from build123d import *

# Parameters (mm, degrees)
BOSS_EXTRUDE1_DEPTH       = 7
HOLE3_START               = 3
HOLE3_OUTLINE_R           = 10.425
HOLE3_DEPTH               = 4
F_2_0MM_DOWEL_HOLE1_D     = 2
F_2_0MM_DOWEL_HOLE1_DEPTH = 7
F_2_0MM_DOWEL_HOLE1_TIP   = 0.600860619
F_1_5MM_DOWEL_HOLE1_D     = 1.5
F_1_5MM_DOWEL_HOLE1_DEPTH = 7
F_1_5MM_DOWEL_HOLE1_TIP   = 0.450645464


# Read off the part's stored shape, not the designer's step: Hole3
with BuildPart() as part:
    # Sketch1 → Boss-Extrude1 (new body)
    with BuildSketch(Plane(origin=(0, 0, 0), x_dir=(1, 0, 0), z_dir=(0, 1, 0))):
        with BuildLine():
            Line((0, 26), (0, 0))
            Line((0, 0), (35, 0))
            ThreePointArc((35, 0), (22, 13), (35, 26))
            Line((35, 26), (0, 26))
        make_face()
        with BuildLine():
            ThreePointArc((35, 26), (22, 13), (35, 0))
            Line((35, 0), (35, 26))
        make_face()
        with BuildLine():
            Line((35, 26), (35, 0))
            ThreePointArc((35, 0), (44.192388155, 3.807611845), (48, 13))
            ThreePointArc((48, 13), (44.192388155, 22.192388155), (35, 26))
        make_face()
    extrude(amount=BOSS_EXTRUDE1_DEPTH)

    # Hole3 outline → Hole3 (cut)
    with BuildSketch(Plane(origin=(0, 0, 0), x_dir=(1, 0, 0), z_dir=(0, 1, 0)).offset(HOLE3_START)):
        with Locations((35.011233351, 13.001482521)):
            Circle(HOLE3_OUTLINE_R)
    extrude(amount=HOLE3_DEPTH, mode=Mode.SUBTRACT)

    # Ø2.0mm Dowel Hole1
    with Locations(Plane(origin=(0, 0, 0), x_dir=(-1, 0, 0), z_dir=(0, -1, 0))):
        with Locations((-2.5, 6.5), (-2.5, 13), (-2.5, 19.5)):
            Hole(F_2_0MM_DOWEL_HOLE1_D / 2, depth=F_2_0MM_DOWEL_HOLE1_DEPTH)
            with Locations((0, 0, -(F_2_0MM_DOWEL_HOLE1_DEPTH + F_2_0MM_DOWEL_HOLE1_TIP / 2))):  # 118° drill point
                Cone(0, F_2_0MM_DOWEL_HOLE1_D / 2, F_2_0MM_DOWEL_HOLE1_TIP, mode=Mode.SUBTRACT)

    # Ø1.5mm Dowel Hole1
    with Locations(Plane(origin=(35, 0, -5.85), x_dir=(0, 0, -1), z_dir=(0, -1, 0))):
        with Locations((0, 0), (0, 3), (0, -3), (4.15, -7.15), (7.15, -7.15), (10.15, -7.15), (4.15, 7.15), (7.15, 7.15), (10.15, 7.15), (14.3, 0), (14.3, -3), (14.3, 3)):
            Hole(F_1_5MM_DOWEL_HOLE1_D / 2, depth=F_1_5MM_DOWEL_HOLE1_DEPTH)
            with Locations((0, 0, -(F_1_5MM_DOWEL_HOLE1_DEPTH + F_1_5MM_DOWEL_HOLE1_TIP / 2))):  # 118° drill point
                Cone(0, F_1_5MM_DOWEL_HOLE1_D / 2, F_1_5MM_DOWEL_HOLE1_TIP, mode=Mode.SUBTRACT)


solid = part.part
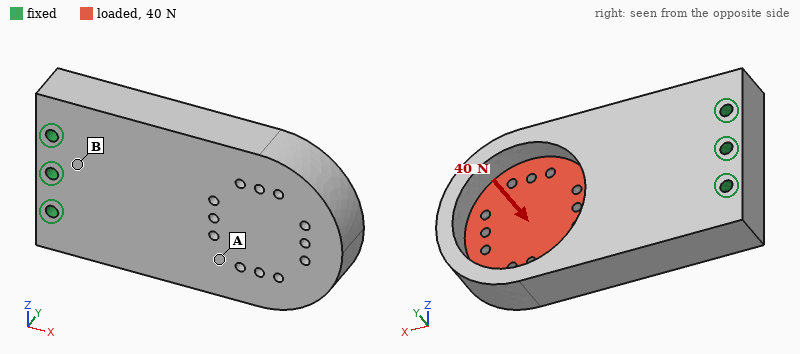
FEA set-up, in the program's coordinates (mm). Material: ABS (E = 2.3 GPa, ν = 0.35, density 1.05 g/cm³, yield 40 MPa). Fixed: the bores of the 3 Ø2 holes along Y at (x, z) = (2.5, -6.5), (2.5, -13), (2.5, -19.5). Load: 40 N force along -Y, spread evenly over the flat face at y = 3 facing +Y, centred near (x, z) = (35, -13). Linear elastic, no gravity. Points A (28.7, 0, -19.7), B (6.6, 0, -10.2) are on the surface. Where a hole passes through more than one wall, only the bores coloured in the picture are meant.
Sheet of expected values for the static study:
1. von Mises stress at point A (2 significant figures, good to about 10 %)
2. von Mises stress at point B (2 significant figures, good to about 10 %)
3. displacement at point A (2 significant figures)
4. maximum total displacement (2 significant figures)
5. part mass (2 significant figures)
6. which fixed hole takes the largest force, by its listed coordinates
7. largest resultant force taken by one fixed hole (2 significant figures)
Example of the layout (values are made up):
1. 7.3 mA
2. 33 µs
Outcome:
1. 2.1 MPa
2. 5.1 MPa
3. 0.22 mm
4. 0.54 mm
5. 7.1 g
6. (2.5, -13)
7. 26 N
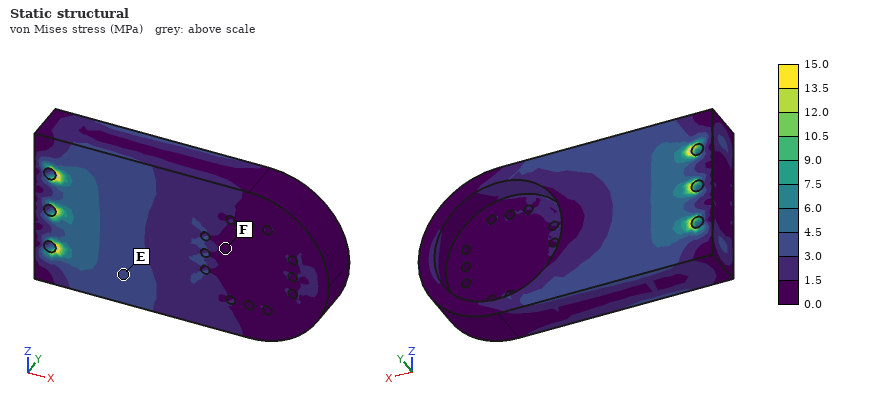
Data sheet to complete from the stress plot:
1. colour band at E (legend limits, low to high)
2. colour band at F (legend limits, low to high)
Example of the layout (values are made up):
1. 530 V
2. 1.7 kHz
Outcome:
1. 3.0 to 4.5 MPa
2. 0.0 to 1.5 MPa
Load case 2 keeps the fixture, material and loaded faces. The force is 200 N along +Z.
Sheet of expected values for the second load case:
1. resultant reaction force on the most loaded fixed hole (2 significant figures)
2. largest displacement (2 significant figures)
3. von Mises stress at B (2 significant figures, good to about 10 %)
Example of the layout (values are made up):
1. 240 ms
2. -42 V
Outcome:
1. 450 N
2. 0.40 mm
3. 6.3 MPa
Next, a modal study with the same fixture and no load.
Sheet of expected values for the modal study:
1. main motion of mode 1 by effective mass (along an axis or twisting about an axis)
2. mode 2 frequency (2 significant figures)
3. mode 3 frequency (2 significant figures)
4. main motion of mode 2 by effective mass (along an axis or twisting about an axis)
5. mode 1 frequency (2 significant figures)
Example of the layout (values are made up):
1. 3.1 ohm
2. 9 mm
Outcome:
1. along Y
2. 2500 Hz
3. 2800 Hz
4. along Z
5. 1000 Hz
